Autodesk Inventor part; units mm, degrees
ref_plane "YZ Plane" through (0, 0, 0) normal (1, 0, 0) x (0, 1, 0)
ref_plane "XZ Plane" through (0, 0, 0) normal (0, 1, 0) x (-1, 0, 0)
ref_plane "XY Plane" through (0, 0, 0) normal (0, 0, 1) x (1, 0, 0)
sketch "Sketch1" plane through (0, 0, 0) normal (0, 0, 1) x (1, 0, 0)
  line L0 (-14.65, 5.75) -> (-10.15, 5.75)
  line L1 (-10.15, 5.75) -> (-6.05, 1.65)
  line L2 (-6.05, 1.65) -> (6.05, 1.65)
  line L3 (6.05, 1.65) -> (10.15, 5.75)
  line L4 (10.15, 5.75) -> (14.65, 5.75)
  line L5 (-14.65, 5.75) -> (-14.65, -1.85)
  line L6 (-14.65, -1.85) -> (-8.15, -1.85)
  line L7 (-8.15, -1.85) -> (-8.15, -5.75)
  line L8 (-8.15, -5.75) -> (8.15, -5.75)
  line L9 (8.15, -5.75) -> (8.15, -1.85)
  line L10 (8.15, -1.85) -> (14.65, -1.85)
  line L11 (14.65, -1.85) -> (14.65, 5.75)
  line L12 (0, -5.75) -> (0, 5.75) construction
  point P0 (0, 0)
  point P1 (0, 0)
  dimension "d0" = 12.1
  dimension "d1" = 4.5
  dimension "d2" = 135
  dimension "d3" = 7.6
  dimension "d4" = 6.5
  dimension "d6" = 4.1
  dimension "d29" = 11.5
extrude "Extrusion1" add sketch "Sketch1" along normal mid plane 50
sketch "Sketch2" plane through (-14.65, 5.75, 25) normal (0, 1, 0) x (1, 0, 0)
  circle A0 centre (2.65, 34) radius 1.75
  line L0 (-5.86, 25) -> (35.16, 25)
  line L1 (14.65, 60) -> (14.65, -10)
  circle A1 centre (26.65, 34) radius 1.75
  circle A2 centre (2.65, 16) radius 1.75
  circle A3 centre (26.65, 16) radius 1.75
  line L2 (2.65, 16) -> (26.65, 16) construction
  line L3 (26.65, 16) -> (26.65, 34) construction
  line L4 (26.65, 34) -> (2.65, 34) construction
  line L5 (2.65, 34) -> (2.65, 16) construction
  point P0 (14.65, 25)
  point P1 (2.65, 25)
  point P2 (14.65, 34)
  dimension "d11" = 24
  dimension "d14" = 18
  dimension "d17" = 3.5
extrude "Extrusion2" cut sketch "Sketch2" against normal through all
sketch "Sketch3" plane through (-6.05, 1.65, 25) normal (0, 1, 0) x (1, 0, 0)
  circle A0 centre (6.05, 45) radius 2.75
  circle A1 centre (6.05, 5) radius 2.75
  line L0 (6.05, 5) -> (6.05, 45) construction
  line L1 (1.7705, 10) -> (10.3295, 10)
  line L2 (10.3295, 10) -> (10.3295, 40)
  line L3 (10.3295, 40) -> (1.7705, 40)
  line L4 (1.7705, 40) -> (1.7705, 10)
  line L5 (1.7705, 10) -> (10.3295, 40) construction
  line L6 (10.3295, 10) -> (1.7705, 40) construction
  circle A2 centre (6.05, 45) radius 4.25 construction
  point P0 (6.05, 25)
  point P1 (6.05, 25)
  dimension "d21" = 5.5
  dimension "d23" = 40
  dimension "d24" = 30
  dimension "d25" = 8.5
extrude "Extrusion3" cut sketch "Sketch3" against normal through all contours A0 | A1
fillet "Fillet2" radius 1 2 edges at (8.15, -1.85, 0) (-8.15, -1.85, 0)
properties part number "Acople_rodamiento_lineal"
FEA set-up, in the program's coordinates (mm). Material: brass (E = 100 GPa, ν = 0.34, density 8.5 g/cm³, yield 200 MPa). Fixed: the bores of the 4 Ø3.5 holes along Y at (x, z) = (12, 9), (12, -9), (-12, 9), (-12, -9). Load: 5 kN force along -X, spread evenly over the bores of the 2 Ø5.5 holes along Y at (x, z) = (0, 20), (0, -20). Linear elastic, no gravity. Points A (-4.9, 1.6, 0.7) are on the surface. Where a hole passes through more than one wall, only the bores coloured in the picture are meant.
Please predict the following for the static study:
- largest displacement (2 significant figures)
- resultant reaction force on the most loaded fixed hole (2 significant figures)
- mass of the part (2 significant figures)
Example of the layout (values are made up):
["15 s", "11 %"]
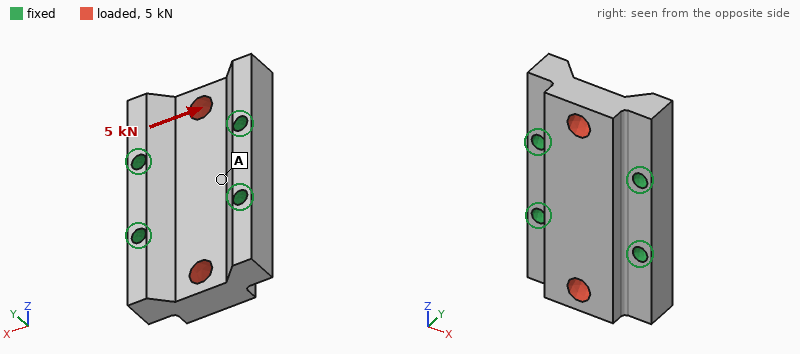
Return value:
["8.9 µm", "1.6 kN", "88 g"]
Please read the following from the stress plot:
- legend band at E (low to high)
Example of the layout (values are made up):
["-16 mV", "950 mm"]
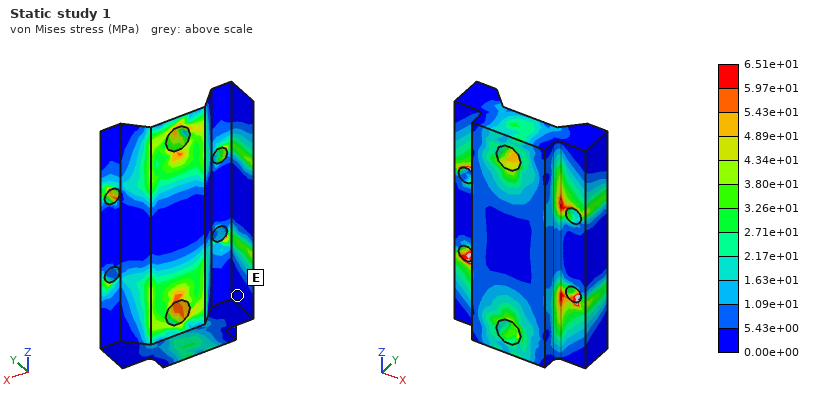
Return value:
["0.00e+00 to 5.43e+00 MPa"]
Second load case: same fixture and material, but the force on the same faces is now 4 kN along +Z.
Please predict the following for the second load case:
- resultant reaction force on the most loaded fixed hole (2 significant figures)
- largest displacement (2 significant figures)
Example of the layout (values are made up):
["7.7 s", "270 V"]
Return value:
["1.0 kN", "9.5 µm"]
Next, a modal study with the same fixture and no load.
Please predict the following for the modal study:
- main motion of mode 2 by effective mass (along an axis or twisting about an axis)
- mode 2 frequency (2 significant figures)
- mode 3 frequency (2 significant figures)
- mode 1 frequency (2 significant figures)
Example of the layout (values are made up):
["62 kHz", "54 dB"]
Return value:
["along Y", "14 kHz", "18 kHz", "13 kHz"]
